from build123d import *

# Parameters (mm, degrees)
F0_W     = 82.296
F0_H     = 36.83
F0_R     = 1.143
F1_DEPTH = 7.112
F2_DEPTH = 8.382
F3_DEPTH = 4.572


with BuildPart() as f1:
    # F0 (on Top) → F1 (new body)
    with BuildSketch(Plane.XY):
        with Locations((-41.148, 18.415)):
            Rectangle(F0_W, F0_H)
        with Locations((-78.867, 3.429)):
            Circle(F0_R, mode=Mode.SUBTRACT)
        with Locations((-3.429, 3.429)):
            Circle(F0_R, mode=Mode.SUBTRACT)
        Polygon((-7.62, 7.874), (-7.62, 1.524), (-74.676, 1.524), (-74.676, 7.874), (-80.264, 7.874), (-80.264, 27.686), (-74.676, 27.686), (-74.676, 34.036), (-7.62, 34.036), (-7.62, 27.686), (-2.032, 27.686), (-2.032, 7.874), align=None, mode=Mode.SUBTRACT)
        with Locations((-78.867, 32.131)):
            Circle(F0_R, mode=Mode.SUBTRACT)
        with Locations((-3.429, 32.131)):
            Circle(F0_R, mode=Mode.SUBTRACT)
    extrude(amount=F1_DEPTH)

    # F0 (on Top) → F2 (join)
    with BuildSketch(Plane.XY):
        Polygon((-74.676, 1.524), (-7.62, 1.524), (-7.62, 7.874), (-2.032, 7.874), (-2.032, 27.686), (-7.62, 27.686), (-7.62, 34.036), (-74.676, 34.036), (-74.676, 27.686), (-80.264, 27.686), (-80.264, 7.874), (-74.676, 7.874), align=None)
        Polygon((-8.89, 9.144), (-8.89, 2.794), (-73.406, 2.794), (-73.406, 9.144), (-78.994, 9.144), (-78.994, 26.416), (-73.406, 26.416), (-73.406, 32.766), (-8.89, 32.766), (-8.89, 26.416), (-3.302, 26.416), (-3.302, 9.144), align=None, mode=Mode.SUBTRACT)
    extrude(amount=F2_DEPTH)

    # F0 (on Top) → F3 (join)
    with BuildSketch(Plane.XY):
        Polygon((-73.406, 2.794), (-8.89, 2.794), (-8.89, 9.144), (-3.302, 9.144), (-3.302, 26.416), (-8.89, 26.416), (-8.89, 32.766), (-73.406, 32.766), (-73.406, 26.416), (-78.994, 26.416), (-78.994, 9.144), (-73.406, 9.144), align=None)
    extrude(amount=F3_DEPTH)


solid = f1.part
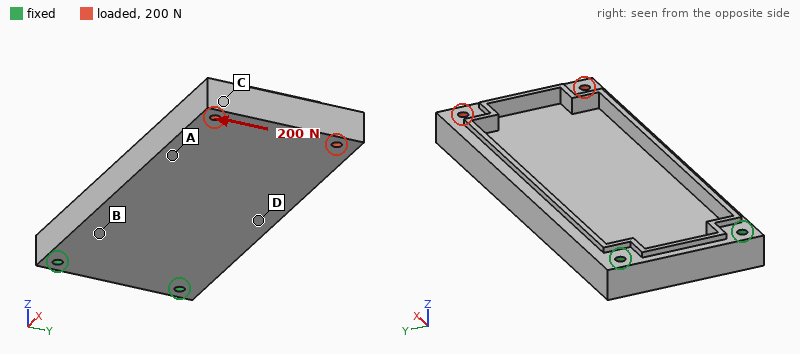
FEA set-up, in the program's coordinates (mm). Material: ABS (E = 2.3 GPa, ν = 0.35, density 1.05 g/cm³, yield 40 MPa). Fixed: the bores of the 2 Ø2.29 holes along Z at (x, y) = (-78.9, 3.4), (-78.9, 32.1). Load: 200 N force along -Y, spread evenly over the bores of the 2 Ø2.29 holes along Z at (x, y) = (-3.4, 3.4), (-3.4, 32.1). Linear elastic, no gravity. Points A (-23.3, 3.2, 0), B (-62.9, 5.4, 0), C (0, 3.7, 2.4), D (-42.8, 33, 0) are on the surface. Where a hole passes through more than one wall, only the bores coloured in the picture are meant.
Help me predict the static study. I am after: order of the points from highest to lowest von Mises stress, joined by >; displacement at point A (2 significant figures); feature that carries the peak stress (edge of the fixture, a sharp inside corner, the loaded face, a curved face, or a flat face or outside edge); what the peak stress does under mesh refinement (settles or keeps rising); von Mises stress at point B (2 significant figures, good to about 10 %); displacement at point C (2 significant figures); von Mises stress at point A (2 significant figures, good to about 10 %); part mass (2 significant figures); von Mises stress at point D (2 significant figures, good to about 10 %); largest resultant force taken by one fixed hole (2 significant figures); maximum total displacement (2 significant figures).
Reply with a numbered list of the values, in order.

1. B > D > A > C
2. 0.48 mm
3. edge of the fixture
4. keeps rising
5. 7.1 MPa
6. 0.79 mm
7. 2.5 MPa
8. 17 g
9. 5.2 MPa
10. 520 N
11. 0.98 mm
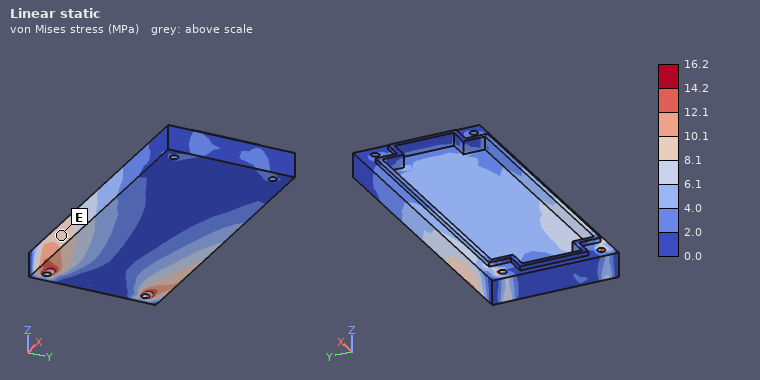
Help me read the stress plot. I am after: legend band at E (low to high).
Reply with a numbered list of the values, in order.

1. 8.1 to 10.1 MPa
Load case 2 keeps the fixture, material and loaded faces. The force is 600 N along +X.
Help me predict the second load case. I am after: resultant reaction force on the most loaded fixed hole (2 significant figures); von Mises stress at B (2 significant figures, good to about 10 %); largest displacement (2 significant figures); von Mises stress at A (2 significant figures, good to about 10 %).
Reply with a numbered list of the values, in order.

1. 310 N
2. 1.6 MPa
3. 1.1 mm
4. 1.7 MPa
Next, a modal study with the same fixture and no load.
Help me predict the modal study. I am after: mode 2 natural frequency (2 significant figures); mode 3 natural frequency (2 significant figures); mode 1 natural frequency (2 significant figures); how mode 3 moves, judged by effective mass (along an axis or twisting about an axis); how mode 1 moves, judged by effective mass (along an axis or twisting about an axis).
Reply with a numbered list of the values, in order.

1. 750 Hz
2. 1200 Hz
3. 210 Hz
4. along Y
5. along Z
